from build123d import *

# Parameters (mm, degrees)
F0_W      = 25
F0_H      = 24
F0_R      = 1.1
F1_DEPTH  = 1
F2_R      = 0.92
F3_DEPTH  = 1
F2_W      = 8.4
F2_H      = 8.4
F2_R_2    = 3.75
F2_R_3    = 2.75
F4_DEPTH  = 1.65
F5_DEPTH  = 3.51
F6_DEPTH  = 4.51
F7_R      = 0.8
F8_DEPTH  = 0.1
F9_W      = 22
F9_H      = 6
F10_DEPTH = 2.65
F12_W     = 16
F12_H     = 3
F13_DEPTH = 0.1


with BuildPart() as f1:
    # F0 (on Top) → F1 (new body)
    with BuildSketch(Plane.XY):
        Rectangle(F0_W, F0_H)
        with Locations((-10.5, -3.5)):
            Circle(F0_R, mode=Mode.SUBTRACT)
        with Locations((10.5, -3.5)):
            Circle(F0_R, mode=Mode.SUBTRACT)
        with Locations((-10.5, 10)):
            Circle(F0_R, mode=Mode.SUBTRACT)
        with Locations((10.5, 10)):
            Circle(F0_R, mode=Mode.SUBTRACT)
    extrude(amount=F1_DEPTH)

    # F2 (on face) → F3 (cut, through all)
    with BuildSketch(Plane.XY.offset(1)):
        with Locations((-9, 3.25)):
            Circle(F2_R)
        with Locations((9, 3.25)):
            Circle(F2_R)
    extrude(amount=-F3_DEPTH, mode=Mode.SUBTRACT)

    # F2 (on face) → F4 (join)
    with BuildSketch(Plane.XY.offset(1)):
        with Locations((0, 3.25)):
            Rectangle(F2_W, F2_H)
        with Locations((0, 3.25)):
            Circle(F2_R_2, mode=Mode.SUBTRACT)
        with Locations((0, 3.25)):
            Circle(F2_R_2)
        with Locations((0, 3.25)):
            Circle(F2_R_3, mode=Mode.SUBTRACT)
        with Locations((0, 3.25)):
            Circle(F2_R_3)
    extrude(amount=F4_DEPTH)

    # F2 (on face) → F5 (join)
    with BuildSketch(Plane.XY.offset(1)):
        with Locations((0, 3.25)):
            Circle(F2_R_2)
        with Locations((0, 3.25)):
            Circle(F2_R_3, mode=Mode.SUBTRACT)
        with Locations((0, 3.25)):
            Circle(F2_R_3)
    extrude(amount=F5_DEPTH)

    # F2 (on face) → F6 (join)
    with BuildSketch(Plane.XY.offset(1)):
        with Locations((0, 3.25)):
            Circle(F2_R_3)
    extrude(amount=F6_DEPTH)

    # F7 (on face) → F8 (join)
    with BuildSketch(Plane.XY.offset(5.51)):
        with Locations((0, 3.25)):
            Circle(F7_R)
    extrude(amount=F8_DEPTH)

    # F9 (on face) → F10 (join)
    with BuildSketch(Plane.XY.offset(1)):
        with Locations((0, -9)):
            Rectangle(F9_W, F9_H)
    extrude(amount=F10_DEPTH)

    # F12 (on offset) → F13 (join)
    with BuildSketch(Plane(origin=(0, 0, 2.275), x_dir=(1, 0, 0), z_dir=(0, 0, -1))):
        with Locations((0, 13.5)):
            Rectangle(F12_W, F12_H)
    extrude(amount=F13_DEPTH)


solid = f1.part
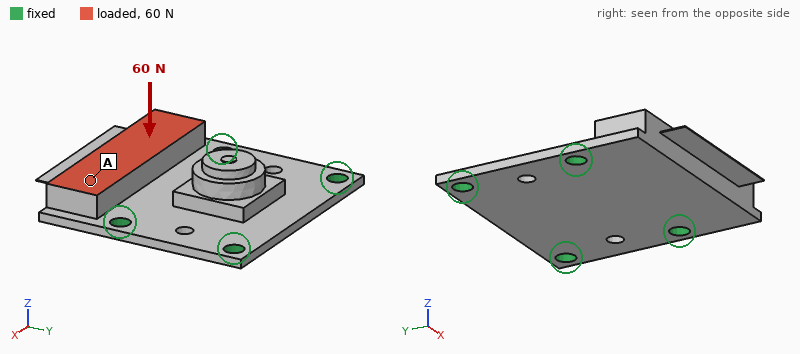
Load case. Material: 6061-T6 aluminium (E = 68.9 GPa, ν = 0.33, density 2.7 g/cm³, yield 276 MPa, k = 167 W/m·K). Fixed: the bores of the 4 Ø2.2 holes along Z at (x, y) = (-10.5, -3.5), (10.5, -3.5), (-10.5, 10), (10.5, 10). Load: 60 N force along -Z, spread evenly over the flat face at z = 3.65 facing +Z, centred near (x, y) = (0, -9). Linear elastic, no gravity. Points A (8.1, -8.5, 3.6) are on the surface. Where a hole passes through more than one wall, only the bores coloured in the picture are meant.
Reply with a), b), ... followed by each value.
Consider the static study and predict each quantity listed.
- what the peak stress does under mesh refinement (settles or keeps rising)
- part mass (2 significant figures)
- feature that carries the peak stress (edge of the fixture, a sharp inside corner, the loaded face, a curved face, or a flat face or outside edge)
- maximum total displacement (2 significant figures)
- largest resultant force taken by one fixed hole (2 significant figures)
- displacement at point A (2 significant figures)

a) keeps rising
b) 3.1 g
c) edge of the fixture
d) 52 µm
e) 39 N
f) 24 µm
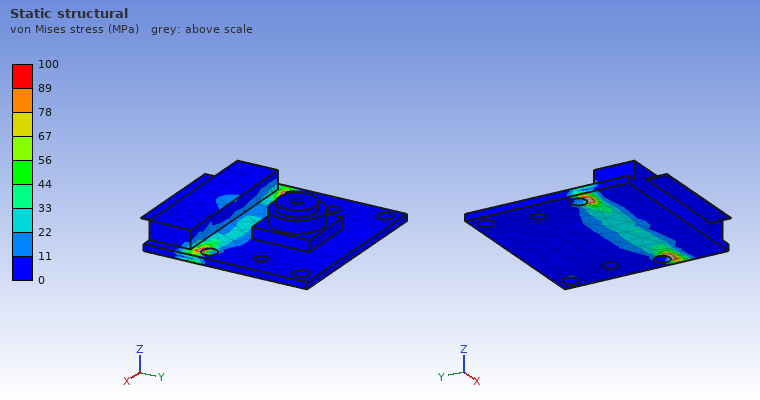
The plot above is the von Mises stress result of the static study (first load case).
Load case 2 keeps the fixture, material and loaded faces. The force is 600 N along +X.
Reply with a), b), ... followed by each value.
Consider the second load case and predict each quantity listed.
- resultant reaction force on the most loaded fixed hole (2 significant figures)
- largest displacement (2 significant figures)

a) 330 N
b) 16 µm
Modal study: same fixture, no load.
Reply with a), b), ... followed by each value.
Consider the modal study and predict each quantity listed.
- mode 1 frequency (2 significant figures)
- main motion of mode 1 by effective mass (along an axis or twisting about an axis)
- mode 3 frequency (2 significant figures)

a) 6200 Hz
b) along Z
c) 11 kHz
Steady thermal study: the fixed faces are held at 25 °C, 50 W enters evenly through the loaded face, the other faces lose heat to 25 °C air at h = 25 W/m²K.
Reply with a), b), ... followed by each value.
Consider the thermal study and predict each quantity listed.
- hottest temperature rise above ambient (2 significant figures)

a) 77 K
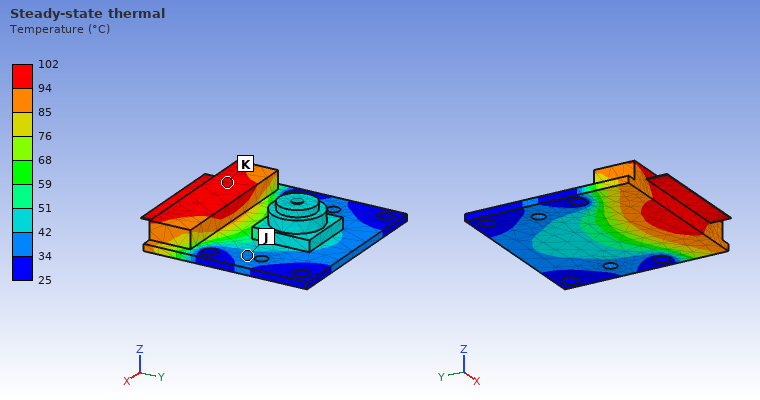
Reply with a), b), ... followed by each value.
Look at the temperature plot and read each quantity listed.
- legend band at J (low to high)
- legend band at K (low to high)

a) 34 to 42 °C
b) 94 to 102 °C
